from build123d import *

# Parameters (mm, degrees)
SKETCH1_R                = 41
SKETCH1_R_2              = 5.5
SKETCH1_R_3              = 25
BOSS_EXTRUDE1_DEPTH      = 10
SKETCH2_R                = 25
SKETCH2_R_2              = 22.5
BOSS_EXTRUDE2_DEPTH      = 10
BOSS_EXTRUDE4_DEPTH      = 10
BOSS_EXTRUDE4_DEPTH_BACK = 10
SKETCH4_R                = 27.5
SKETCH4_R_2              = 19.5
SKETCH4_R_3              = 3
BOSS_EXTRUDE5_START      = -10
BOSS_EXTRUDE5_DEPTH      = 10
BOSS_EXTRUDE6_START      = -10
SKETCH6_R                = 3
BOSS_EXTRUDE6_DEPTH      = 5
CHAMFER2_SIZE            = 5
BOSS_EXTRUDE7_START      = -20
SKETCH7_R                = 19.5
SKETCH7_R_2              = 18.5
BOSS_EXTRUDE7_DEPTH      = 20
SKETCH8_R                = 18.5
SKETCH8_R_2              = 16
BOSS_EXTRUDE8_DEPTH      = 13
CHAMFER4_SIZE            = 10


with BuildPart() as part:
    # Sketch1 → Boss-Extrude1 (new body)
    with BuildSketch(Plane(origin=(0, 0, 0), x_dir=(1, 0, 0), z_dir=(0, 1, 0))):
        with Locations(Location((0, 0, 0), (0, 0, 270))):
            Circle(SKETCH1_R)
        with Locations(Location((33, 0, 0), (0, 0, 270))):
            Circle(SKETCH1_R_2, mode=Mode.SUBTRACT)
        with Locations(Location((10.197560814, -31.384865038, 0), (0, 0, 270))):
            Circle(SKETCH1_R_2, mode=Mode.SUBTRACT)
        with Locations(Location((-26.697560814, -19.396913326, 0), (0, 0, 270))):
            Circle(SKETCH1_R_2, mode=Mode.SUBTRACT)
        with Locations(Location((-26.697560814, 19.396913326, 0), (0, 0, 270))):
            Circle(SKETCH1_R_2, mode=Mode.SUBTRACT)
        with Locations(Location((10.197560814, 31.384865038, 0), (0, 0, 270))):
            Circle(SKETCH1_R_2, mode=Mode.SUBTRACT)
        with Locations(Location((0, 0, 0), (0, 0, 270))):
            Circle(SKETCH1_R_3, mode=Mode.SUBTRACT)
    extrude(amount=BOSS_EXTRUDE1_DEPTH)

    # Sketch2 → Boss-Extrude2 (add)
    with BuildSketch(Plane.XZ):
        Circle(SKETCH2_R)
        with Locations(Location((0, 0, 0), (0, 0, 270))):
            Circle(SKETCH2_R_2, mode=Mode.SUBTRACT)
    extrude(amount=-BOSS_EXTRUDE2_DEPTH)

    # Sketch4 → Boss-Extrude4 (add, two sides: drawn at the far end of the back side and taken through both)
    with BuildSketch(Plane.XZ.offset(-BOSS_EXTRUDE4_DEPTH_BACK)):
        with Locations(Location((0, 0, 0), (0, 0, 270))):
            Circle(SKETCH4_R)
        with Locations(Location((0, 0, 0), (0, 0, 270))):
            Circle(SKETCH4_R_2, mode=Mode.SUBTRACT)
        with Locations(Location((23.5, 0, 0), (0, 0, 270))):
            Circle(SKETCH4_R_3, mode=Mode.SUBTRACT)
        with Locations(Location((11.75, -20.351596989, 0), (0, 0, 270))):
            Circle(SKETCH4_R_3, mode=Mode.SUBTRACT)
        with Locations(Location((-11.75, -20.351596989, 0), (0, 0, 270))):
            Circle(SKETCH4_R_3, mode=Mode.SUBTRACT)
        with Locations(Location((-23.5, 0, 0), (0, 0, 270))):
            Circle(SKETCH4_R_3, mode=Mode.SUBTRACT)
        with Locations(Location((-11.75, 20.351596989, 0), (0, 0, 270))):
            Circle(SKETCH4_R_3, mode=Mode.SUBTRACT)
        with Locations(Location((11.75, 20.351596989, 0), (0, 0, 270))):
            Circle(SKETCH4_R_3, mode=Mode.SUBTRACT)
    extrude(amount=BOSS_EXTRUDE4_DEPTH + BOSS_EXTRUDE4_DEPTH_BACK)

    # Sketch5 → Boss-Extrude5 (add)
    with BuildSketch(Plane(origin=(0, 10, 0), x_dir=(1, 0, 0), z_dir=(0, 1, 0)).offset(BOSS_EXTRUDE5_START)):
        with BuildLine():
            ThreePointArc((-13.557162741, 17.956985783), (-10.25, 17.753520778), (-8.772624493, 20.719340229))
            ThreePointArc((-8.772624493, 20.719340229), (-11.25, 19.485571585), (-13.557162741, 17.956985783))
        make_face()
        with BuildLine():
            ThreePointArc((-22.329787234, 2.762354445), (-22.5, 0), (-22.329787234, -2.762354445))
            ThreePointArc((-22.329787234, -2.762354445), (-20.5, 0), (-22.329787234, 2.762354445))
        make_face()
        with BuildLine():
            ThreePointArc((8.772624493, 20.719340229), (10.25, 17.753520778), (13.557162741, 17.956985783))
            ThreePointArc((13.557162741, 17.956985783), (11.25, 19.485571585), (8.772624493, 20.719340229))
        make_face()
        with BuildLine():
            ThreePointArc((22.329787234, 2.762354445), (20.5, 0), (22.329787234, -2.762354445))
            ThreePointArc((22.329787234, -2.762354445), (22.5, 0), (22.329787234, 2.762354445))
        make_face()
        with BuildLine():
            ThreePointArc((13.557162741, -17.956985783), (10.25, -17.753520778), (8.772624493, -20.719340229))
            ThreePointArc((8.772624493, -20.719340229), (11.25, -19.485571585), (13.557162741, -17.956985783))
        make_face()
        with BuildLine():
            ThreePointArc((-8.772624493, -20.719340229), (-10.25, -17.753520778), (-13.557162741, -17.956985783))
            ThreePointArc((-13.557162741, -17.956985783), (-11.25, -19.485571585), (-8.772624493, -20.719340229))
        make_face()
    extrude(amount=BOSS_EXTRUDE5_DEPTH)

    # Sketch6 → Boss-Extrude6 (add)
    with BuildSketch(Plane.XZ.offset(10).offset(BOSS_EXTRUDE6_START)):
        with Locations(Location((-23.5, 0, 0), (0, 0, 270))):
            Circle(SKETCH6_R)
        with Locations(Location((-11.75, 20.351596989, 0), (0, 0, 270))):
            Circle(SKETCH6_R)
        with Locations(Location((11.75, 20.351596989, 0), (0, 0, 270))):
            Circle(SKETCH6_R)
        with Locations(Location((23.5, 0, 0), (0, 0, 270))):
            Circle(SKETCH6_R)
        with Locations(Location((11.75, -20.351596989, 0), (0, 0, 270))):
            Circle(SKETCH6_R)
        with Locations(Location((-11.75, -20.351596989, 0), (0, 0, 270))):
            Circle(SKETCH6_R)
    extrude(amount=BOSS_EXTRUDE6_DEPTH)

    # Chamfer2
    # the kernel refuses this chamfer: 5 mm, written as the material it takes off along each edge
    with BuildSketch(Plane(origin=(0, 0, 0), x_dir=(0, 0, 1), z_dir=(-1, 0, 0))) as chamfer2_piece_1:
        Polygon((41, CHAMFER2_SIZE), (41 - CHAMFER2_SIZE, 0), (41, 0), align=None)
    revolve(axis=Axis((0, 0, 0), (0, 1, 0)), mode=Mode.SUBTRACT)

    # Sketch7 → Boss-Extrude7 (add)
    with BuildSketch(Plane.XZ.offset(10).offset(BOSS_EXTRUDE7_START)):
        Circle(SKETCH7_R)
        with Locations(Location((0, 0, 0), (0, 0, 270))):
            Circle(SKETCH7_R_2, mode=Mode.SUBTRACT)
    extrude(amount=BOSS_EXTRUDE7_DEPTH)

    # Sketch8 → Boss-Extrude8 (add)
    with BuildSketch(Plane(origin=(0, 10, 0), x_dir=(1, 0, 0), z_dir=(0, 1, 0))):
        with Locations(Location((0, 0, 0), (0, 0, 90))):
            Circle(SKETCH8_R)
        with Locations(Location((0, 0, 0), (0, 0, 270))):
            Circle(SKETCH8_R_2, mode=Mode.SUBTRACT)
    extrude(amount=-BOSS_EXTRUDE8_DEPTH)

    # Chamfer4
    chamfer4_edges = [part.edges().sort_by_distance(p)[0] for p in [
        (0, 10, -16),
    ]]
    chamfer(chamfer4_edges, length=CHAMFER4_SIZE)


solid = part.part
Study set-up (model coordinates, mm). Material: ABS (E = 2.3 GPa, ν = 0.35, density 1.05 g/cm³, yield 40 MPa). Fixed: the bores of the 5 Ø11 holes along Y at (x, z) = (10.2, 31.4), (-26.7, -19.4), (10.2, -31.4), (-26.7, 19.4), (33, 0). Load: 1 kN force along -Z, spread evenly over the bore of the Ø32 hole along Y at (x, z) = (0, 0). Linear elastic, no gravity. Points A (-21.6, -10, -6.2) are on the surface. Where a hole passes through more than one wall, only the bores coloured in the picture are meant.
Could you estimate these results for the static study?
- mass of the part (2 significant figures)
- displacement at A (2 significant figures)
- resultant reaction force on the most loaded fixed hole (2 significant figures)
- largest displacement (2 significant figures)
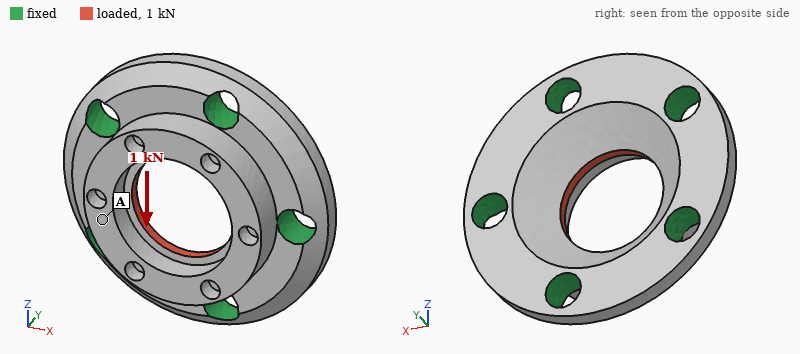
46 g
7.4 µm
240 N
25 µm
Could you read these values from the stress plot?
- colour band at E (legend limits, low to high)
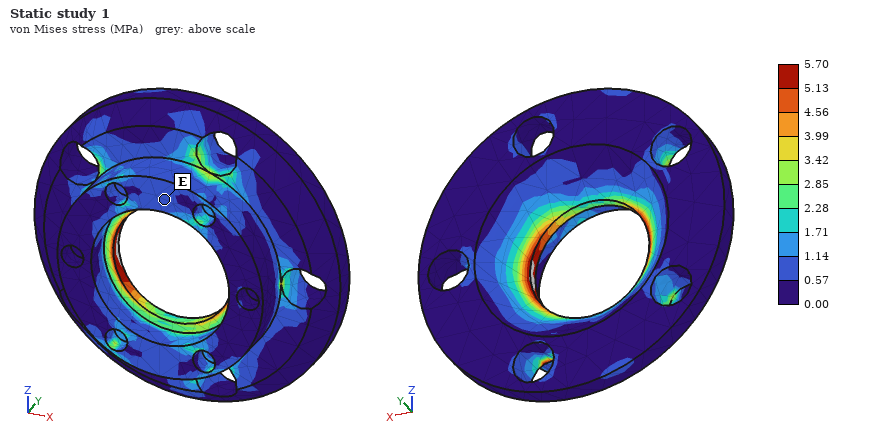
0.57 to 1.14 MPa
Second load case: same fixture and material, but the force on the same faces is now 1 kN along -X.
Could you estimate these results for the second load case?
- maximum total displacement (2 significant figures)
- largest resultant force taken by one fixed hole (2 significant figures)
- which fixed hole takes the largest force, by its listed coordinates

26 µm
250 N
(33, 0)
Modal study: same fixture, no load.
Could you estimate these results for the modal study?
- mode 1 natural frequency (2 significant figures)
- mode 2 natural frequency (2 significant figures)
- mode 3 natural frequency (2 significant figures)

8400 Hz
8700 Hz
8800 Hz
